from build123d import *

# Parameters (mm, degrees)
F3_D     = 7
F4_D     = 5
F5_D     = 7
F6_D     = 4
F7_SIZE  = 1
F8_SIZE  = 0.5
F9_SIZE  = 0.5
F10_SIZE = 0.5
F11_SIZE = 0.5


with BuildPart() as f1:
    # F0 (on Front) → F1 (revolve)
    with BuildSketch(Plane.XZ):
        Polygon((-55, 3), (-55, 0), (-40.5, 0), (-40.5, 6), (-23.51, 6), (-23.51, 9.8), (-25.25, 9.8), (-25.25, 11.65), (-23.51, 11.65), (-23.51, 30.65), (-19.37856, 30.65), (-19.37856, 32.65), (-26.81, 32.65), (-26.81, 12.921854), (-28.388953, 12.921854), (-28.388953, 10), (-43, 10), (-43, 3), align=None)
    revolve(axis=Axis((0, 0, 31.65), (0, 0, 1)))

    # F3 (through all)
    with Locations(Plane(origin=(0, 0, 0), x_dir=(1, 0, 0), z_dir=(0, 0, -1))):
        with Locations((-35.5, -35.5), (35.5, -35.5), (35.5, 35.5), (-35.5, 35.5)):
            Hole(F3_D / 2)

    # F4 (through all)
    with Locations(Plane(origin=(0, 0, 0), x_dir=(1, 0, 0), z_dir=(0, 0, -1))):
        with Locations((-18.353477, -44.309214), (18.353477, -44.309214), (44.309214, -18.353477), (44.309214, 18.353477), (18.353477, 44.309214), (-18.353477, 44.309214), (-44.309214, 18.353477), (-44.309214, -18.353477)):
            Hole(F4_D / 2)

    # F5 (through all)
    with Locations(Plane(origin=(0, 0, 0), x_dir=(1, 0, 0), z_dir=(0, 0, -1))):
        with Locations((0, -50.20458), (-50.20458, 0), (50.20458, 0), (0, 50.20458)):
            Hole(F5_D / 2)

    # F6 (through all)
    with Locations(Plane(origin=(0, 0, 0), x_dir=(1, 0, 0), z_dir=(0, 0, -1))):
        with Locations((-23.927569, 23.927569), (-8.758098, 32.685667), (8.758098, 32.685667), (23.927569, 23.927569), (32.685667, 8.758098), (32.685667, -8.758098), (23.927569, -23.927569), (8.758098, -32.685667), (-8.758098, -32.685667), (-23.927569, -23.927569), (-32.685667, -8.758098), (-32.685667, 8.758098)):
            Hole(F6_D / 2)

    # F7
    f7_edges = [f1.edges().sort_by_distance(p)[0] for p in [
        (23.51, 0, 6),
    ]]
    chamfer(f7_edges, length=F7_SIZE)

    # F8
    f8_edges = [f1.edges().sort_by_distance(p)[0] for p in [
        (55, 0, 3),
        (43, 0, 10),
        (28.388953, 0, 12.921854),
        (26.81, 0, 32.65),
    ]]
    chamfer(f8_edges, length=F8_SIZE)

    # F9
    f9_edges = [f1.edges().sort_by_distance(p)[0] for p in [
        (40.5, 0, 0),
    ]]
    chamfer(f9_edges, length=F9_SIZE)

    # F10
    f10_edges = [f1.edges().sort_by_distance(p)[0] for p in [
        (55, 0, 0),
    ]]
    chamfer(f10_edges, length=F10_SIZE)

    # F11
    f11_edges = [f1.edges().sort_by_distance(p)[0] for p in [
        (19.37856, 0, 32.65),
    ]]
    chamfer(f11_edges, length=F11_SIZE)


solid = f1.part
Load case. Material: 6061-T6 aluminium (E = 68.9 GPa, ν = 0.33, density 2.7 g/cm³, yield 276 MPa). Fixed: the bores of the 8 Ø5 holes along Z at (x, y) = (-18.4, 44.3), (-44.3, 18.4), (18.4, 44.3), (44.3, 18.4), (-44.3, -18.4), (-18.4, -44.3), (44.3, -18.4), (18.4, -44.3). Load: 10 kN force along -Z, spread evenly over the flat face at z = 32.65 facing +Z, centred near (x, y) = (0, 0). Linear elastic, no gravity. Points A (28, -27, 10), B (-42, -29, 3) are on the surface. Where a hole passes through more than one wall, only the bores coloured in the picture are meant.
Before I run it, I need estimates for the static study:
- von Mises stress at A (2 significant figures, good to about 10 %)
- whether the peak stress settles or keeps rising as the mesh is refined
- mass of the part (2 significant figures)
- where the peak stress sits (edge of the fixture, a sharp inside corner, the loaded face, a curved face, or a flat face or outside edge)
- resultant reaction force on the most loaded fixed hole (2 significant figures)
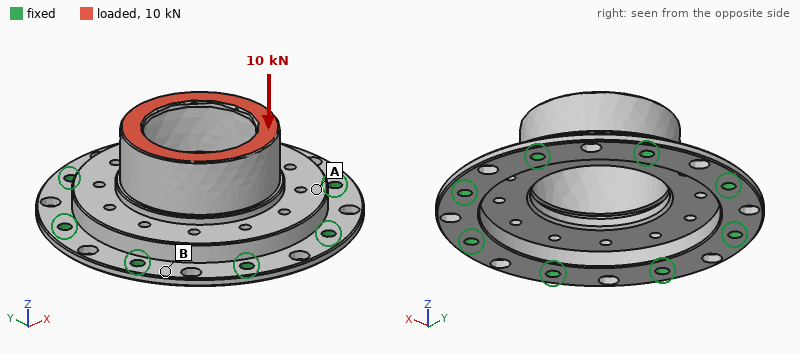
58 MPa
keeps rising
110 g
edge of the fixture
2.3 kN
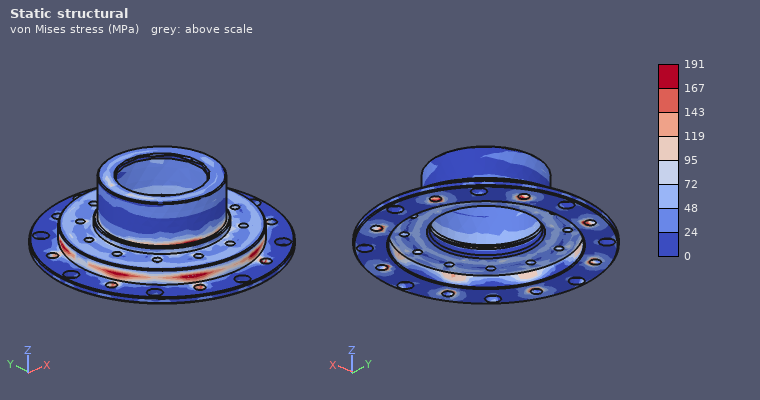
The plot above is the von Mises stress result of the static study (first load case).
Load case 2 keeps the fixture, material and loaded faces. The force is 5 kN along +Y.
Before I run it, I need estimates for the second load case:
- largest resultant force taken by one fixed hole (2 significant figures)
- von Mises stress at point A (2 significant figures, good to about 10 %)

1.4 kN
25 MPa
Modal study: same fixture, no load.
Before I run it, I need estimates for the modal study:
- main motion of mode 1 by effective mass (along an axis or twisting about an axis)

along Z
